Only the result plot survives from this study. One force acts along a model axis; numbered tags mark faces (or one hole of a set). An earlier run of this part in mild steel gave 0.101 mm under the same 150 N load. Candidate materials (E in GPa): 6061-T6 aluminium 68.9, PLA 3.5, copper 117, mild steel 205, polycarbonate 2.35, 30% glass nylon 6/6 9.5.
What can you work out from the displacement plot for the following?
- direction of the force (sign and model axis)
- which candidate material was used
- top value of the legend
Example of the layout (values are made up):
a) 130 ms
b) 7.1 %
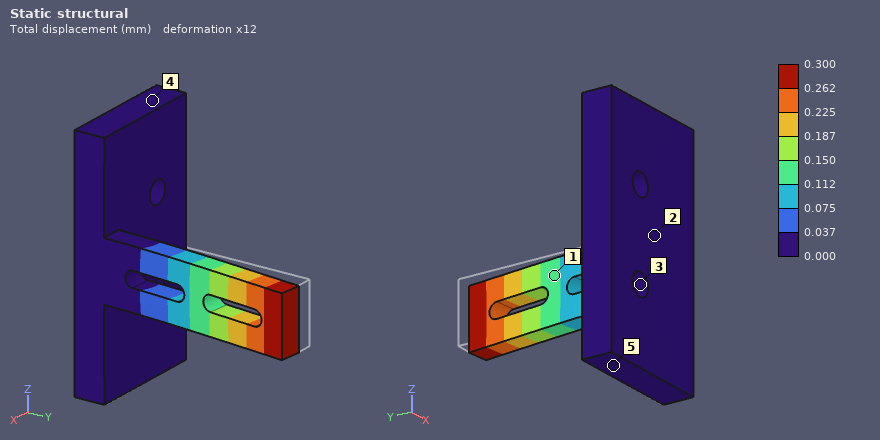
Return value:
a) +X
b) 6061-T6 aluminium
c) 0.300 mm
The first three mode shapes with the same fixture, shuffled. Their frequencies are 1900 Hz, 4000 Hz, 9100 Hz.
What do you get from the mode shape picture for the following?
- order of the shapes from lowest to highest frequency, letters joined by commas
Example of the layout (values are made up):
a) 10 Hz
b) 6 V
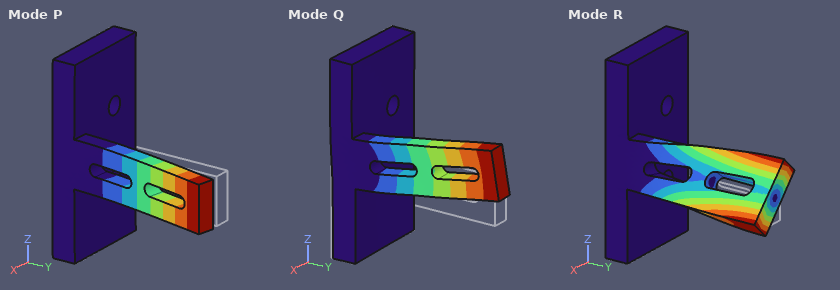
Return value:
a) P, Q, R
